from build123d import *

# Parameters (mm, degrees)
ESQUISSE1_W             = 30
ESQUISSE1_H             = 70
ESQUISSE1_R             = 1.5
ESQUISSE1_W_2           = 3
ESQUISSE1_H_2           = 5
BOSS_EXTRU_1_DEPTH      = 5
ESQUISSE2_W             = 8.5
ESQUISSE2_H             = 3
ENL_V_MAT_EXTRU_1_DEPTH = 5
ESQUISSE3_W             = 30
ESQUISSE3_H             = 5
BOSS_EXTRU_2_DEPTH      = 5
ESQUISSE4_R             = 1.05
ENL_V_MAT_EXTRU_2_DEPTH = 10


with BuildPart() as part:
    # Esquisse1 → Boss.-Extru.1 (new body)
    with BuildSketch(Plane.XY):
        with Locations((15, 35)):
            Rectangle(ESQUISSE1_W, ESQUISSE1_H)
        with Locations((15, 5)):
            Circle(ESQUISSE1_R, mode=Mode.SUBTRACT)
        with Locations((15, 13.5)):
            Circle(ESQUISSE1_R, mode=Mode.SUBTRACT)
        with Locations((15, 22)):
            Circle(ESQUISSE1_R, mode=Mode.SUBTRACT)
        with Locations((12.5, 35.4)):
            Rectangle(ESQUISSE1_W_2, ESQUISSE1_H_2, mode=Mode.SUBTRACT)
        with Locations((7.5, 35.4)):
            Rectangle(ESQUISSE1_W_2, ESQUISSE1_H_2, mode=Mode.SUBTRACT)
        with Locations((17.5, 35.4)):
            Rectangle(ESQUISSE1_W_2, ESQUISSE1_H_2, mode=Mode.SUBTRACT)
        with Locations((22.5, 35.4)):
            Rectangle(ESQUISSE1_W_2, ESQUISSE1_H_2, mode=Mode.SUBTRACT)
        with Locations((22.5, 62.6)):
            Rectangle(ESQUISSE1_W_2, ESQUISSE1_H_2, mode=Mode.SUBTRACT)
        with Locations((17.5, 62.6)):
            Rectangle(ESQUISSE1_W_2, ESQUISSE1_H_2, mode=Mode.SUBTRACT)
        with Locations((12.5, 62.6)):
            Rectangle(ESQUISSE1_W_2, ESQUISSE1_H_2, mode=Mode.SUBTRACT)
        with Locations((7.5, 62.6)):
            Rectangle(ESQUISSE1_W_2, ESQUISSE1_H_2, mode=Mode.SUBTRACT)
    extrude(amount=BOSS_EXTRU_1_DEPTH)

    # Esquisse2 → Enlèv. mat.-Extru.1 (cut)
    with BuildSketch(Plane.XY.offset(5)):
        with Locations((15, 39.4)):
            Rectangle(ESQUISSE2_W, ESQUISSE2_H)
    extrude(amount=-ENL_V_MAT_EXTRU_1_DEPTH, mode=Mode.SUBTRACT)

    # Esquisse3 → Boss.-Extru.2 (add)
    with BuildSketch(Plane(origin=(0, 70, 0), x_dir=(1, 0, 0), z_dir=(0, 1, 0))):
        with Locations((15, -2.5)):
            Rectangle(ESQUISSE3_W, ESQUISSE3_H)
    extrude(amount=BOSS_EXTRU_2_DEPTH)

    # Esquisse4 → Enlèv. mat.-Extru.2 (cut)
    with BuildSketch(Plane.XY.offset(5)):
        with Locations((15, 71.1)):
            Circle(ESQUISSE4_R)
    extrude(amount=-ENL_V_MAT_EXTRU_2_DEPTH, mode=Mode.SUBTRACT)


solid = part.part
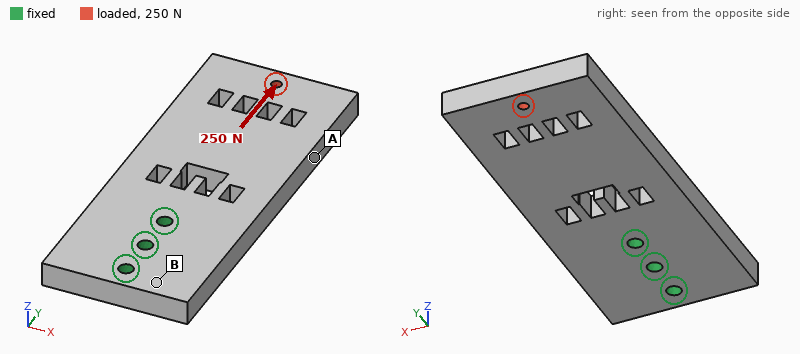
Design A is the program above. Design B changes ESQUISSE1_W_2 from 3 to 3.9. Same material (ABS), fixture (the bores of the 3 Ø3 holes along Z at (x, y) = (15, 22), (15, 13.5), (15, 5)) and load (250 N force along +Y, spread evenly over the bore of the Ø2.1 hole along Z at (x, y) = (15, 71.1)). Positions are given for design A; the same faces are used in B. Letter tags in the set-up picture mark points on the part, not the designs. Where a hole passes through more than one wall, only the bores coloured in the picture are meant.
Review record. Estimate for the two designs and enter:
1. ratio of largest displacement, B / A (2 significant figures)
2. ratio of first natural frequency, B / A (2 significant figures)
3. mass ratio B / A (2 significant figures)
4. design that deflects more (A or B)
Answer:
1.2
0.97
0.98
B
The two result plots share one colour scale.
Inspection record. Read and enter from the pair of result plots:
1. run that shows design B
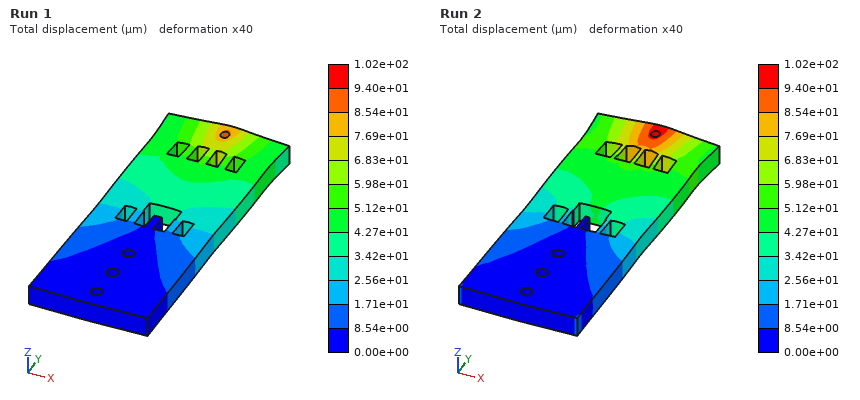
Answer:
Run 2
